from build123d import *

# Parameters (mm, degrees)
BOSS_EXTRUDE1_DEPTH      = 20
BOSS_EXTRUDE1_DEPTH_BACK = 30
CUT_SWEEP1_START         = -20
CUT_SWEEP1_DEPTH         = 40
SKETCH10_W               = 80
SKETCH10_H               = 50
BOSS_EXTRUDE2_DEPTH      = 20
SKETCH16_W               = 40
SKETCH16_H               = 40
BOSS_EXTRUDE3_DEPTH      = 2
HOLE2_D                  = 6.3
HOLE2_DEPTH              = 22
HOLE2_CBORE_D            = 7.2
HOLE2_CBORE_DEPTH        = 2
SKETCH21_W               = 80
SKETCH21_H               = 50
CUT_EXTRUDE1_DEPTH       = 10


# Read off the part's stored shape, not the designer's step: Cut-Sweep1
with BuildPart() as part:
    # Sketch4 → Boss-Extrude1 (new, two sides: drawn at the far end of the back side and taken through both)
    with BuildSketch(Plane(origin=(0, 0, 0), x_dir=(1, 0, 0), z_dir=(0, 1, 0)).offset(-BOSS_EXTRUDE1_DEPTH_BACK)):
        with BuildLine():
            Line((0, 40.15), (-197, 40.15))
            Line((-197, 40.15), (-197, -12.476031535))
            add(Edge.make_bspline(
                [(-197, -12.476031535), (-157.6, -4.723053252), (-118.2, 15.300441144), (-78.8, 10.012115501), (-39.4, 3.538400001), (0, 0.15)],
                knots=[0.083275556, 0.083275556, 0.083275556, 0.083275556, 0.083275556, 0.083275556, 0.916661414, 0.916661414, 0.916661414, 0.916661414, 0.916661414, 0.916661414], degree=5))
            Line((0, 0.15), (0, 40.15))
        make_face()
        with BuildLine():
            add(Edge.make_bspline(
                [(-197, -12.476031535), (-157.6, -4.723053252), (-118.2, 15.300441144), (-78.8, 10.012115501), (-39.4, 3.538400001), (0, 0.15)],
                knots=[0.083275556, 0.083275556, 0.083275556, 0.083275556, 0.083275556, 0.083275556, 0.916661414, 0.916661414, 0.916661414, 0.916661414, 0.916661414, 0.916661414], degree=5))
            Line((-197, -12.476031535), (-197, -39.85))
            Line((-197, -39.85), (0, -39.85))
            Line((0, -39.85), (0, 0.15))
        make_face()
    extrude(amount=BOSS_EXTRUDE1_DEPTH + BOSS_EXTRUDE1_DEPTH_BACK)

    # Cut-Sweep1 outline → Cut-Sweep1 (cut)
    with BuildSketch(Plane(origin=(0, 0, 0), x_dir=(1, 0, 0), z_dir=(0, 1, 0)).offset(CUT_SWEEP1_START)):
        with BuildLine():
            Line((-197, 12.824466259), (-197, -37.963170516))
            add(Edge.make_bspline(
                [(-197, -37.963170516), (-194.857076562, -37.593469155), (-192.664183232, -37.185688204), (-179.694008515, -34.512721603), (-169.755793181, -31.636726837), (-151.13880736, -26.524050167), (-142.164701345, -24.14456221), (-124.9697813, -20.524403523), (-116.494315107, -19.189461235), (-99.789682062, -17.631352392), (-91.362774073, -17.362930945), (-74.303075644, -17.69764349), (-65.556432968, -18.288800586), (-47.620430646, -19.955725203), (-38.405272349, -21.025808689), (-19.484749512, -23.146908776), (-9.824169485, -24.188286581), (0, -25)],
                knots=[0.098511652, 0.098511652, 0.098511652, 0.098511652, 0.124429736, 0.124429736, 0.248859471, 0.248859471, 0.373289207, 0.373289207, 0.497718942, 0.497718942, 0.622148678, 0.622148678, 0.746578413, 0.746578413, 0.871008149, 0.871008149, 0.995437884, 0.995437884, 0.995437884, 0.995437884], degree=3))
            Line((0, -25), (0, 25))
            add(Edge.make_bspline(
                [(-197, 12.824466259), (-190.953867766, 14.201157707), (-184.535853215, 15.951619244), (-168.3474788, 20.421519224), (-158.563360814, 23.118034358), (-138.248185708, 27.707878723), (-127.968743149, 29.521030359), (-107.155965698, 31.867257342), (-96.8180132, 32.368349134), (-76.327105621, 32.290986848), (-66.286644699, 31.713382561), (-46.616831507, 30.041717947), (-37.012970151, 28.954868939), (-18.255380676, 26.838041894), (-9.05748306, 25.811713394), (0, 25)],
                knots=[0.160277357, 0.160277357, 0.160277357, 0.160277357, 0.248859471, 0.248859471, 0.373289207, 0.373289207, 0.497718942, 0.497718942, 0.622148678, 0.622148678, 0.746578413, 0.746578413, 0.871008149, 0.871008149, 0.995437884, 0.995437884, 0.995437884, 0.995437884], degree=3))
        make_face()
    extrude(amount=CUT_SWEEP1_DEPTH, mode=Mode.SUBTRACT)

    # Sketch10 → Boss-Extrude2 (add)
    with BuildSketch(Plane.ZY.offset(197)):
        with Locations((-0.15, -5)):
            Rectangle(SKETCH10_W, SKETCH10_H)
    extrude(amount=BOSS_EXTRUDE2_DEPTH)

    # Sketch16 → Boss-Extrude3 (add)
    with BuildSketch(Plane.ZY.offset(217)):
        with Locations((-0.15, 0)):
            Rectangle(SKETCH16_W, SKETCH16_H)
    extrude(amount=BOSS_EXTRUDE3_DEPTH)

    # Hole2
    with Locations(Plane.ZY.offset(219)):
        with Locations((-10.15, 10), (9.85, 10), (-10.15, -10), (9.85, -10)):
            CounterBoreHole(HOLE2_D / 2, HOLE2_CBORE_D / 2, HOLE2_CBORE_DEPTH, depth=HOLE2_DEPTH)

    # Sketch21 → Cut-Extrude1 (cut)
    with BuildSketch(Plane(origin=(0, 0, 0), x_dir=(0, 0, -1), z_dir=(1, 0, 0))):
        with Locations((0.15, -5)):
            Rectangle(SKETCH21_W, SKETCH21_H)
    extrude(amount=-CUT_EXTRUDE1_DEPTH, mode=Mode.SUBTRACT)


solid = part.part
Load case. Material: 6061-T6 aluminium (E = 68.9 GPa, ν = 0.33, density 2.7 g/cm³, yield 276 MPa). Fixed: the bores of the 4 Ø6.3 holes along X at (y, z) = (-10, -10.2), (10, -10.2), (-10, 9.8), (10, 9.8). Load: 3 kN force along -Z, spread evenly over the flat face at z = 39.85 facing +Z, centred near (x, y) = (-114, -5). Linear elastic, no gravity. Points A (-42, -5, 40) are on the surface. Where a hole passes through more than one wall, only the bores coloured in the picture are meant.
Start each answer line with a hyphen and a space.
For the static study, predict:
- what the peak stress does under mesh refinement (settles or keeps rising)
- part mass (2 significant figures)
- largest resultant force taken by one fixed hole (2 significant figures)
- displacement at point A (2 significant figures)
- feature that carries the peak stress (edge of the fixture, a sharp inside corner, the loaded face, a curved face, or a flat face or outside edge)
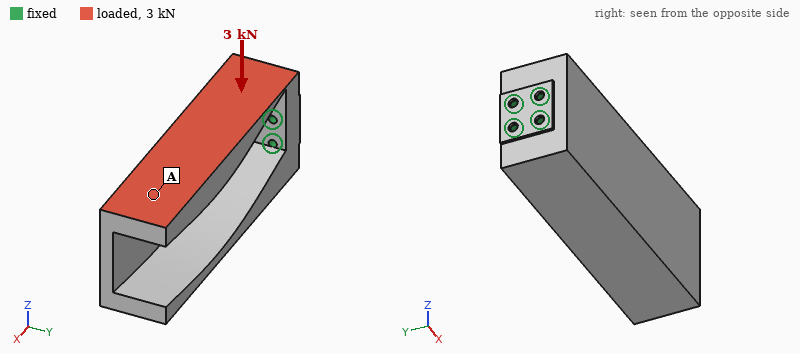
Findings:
- keeps rising
- 1.2 kg
- 5.0 kN
- 0.23 mm
- edge of the fixture
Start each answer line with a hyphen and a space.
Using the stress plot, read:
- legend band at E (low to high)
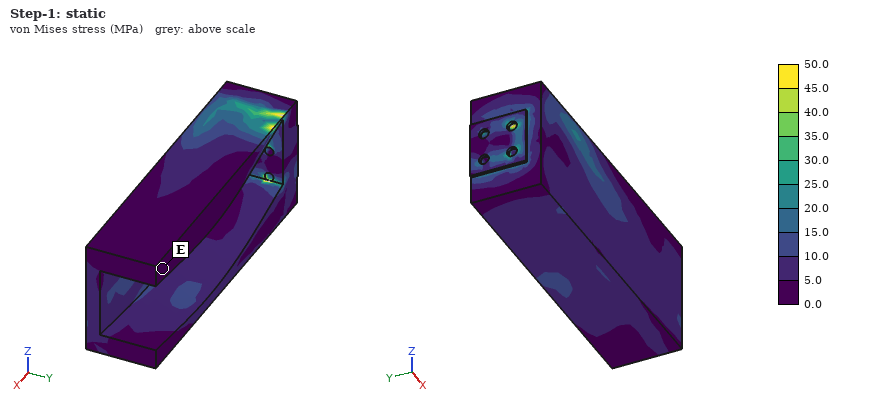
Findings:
- 0.0 to 5.0 MPa
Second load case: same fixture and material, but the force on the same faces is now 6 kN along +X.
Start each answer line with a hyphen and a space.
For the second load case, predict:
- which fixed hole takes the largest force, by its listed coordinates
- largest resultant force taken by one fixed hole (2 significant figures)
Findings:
- (-10, 9.8)
- 5.1 kN
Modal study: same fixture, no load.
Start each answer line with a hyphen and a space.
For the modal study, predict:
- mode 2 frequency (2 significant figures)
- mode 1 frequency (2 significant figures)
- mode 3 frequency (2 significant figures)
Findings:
- 750 Hz
- 560 Hz
- 1500 Hz
